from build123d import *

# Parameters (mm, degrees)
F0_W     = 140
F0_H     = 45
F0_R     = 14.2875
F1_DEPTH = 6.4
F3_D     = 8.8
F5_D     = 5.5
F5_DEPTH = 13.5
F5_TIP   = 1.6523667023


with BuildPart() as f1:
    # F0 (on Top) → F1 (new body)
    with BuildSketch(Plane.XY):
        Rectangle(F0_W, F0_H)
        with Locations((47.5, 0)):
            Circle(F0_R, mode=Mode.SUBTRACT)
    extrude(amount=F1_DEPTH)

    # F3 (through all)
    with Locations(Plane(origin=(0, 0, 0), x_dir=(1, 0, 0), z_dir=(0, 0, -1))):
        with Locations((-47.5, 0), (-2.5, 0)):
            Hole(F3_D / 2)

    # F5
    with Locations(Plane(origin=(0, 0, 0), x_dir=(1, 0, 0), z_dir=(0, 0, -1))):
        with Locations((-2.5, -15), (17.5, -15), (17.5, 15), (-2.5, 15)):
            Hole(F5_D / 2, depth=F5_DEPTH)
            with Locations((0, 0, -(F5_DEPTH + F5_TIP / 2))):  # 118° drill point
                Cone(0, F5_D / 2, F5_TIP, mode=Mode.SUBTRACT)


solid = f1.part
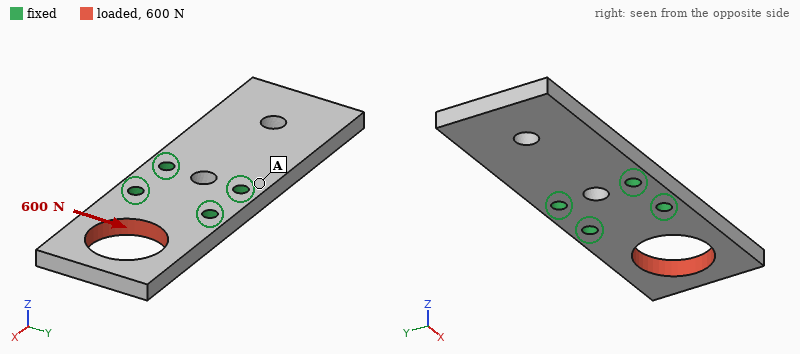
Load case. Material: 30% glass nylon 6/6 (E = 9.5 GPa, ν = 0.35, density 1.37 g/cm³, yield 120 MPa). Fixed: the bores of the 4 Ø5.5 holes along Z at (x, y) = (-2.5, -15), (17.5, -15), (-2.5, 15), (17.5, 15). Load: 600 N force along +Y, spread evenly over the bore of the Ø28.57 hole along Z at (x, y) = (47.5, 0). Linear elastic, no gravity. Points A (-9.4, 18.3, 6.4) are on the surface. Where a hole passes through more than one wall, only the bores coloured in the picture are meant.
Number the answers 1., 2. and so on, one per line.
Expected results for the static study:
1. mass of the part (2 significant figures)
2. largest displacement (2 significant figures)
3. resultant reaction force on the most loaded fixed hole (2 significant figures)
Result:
1. 48 g
2. 0.14 mm
3. 550 N
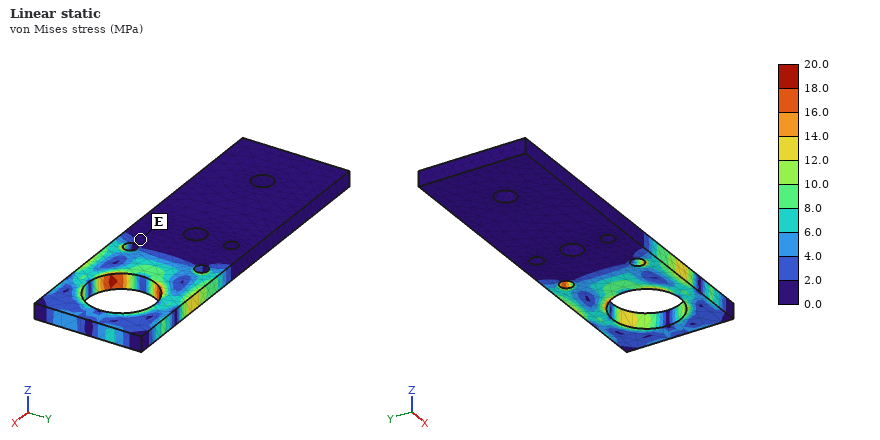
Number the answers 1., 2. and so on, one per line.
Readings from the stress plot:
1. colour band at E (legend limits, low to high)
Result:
1. 0.0 to 2.0 MPa
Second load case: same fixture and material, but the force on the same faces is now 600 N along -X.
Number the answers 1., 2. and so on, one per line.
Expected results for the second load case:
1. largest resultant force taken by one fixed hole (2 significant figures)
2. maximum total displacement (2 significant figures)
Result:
1. 270 N
2. 29 µm
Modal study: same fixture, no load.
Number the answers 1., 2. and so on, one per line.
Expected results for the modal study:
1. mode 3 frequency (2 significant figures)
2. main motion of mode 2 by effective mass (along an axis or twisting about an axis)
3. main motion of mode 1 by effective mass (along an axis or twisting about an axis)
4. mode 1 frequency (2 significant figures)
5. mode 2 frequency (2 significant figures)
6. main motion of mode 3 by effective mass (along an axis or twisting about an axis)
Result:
1. 1900 Hz
2. along Z
3. along Z
4. 600 Hz
5. 950 Hz
6. twisting about X
